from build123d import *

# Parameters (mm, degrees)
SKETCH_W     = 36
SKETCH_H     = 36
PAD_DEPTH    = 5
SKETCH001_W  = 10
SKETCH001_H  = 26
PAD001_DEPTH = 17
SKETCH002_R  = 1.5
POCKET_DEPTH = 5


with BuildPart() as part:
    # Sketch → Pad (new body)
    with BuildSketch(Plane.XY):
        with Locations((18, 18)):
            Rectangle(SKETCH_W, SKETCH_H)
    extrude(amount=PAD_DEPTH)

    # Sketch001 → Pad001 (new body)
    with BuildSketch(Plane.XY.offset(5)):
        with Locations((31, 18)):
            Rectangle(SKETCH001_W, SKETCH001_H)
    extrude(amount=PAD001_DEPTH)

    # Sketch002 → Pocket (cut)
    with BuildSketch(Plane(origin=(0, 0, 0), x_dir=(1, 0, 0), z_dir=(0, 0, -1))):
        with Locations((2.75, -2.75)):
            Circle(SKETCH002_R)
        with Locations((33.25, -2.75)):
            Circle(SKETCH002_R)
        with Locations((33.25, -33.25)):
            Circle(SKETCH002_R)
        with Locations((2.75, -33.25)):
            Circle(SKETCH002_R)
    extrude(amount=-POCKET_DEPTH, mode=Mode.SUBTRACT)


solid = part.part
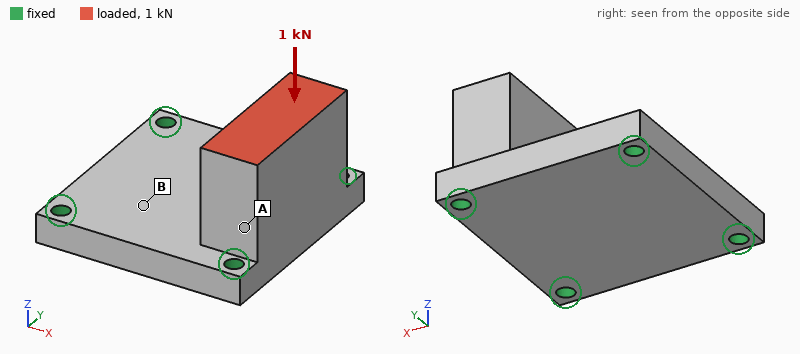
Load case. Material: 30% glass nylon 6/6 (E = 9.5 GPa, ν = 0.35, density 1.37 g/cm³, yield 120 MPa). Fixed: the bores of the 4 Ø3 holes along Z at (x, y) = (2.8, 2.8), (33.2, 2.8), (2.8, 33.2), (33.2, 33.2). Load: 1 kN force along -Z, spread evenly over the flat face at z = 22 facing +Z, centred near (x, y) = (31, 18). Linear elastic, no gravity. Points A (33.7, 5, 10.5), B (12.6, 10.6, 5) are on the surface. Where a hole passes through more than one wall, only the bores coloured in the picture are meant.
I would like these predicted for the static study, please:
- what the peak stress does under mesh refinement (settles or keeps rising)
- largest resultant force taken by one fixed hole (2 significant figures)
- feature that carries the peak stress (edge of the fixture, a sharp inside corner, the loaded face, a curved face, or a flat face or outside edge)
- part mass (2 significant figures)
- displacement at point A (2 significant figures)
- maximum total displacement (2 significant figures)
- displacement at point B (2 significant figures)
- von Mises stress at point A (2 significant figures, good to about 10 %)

keeps rising
500 N
edge of the fixture
15 g
19 µm
31 µm
13 µm
8.0 MPa
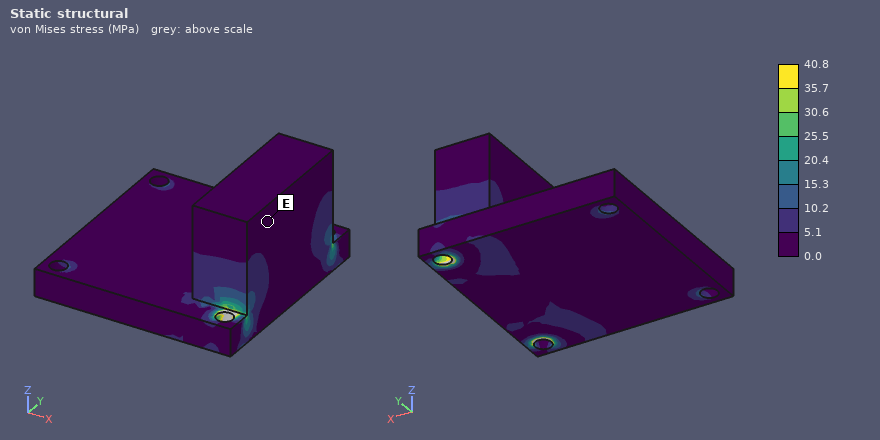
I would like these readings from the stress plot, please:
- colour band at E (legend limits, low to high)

0.0 to 5.1 MPa
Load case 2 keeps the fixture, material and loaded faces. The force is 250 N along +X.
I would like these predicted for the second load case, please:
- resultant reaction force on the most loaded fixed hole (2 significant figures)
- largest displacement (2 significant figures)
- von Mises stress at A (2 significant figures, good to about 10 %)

120 N
0.11 mm
5.8 MPa
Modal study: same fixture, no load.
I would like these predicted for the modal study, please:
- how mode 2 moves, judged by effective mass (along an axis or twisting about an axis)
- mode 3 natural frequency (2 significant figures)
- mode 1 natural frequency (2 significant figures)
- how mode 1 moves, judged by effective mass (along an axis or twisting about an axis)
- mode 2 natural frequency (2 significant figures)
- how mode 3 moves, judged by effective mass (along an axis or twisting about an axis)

along Z
11 kHz
4800 Hz
along X
10 kHz
along Y
